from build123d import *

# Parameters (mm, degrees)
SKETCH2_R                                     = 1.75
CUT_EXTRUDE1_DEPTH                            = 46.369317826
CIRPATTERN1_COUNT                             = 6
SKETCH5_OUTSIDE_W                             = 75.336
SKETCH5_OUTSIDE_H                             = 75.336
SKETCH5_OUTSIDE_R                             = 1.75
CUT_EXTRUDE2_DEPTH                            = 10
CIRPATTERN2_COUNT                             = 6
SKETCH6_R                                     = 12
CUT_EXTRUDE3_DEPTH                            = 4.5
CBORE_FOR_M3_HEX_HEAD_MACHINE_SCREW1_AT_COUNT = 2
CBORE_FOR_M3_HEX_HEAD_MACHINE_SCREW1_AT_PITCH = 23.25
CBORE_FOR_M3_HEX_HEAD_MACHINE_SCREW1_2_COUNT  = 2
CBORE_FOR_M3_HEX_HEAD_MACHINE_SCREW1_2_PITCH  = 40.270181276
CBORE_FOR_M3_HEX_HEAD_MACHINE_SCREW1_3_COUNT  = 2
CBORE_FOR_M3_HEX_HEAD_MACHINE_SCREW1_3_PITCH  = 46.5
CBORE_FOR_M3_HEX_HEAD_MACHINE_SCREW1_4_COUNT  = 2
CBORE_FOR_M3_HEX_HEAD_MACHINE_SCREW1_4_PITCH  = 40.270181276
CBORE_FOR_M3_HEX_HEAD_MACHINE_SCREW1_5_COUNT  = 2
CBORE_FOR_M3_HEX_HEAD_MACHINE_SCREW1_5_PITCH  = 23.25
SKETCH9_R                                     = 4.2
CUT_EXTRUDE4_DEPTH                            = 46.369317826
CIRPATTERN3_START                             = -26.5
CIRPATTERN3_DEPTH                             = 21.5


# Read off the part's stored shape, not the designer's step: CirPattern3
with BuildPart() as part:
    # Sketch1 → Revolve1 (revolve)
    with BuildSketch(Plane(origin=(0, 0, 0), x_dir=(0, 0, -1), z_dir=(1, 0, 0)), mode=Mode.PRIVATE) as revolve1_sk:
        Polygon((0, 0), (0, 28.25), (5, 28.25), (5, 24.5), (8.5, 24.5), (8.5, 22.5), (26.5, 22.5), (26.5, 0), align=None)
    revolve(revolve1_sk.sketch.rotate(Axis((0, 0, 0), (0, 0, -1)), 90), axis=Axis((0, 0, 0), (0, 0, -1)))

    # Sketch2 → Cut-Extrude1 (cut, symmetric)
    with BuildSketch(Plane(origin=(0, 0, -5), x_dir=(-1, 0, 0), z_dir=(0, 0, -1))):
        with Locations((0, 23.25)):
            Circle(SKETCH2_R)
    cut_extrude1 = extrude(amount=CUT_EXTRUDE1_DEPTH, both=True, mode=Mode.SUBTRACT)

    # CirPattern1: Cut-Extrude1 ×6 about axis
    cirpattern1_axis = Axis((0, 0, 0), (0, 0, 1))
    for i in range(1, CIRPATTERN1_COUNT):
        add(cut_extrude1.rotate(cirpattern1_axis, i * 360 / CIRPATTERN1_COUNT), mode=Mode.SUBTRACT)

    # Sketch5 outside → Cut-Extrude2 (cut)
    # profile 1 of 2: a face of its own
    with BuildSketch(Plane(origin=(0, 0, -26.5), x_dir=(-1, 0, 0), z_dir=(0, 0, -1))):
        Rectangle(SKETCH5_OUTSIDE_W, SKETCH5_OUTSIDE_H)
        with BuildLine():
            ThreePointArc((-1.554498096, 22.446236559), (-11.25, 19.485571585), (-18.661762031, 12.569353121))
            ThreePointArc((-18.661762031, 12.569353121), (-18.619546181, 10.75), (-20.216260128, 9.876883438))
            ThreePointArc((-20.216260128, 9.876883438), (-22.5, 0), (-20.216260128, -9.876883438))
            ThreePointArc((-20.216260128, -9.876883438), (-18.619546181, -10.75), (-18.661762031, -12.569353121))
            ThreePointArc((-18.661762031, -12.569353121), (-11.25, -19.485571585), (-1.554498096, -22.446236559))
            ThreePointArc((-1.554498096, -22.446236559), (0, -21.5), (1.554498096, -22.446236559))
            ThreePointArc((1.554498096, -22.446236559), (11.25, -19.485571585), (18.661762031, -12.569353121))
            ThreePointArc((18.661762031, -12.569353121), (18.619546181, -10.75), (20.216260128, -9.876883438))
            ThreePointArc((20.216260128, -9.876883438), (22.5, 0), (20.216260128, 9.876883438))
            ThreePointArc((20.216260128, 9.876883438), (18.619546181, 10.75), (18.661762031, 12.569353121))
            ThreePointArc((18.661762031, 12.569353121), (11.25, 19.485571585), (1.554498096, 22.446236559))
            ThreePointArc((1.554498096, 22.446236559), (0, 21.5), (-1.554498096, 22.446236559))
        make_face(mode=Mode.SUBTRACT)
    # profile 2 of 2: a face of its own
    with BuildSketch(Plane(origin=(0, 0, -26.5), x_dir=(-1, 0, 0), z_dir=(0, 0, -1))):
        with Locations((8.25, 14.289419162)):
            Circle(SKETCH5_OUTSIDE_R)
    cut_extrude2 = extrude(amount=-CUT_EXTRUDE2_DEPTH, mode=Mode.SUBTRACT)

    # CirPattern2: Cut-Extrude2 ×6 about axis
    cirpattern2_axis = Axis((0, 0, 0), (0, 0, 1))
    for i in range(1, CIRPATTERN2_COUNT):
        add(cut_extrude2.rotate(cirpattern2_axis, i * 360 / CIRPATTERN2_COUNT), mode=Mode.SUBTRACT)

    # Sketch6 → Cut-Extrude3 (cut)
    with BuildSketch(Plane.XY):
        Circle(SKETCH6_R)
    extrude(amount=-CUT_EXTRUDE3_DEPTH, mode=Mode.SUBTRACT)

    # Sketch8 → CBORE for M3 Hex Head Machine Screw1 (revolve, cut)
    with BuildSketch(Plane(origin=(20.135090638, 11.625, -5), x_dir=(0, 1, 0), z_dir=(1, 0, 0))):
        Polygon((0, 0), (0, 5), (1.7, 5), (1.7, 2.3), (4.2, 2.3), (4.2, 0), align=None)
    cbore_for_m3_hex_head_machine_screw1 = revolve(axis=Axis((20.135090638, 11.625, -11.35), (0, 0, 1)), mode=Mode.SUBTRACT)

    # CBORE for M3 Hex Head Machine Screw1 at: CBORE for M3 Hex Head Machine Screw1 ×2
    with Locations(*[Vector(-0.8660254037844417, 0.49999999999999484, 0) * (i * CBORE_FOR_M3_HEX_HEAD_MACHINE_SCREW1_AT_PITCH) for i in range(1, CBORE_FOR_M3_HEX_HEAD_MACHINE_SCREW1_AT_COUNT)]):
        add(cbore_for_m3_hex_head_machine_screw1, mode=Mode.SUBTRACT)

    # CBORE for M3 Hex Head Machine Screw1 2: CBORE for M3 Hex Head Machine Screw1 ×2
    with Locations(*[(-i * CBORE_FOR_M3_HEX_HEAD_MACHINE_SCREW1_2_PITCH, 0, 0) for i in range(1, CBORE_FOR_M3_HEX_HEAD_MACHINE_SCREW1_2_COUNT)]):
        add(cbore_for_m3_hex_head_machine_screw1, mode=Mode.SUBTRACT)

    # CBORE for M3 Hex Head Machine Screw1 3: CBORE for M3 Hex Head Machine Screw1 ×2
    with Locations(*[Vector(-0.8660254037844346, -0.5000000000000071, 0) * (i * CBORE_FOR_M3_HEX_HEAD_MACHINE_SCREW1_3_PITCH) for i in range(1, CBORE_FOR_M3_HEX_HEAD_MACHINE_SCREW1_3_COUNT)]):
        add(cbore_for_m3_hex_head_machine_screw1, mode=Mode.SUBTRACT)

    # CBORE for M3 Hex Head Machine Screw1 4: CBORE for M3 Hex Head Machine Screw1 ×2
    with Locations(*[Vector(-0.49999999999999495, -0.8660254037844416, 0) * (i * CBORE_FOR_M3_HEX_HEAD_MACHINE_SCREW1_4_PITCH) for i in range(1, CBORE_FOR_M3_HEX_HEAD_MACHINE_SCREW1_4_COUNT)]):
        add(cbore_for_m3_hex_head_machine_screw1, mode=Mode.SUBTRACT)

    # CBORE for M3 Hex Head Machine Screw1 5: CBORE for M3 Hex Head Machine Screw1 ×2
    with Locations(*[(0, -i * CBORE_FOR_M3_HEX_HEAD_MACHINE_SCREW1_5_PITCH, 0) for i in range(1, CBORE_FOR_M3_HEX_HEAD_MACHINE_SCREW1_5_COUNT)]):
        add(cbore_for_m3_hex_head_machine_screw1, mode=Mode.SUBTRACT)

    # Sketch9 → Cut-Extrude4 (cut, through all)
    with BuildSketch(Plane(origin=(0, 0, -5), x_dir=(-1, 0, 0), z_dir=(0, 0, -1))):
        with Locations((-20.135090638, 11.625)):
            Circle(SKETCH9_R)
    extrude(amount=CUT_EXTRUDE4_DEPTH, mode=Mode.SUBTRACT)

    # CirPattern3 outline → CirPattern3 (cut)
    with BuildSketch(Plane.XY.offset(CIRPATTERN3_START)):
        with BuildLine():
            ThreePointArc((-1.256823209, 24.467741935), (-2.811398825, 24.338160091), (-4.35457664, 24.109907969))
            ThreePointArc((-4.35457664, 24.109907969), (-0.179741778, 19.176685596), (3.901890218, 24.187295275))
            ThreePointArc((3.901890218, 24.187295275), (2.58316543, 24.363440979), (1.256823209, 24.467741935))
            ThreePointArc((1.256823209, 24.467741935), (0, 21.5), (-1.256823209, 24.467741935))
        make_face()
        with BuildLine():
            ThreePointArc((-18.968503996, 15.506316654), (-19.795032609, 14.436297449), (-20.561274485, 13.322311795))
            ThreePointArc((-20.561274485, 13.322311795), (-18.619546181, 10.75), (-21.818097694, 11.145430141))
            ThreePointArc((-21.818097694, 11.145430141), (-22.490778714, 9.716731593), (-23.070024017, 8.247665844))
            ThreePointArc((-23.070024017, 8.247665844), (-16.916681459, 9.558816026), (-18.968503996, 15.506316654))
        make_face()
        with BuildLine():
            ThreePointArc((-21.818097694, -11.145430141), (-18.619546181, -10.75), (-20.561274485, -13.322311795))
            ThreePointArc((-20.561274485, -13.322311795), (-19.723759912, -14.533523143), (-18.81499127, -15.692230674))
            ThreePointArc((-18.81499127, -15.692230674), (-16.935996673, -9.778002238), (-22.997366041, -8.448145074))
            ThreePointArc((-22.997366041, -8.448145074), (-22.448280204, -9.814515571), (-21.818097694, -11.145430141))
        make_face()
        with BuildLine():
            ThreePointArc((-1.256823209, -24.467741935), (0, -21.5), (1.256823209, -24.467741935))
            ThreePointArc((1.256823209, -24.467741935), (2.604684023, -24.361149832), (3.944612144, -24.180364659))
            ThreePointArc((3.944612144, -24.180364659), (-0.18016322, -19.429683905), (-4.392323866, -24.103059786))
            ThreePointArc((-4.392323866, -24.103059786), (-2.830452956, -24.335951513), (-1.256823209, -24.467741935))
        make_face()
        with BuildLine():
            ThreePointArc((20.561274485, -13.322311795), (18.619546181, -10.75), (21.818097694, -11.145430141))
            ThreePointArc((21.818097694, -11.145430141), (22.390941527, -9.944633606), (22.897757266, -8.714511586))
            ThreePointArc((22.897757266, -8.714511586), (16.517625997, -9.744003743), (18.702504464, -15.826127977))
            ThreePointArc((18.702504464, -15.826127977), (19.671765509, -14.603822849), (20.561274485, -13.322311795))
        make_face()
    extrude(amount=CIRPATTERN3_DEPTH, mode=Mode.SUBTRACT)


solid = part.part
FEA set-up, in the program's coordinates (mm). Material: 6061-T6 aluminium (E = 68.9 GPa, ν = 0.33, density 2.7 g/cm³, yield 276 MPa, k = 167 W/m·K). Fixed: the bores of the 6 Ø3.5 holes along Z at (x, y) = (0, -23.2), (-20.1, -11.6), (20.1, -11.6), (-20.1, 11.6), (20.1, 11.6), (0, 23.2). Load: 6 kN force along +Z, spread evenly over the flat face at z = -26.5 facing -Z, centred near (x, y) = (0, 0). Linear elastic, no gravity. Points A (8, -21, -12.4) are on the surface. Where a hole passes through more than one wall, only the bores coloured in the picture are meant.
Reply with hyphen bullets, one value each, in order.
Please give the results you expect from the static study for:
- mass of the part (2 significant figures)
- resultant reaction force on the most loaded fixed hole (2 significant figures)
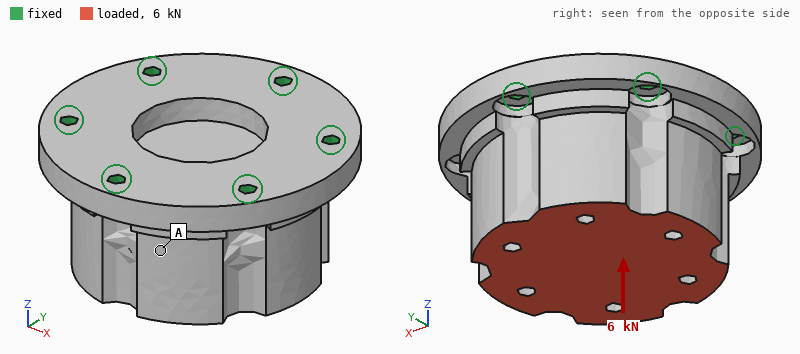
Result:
- 110 g
- 1.1 kN
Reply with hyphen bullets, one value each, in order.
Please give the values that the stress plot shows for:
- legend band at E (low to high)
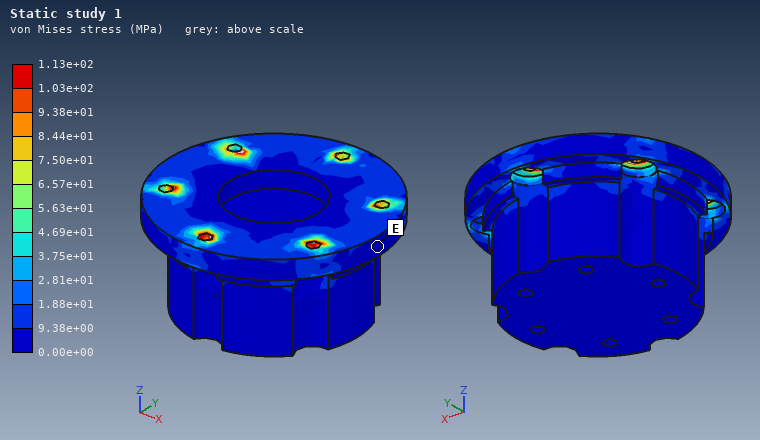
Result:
- 0.00e+00 to 9.38e+00 MPa
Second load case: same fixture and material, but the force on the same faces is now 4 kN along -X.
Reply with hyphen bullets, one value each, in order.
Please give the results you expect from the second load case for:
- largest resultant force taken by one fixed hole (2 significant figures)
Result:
- 1.5 kN
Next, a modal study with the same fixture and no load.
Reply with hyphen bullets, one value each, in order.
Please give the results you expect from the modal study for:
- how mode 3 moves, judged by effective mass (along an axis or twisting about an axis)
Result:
- along Z
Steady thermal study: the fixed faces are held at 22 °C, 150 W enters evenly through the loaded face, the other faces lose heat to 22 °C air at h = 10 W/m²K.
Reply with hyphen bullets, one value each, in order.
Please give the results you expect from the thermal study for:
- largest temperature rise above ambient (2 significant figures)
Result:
- 31 K
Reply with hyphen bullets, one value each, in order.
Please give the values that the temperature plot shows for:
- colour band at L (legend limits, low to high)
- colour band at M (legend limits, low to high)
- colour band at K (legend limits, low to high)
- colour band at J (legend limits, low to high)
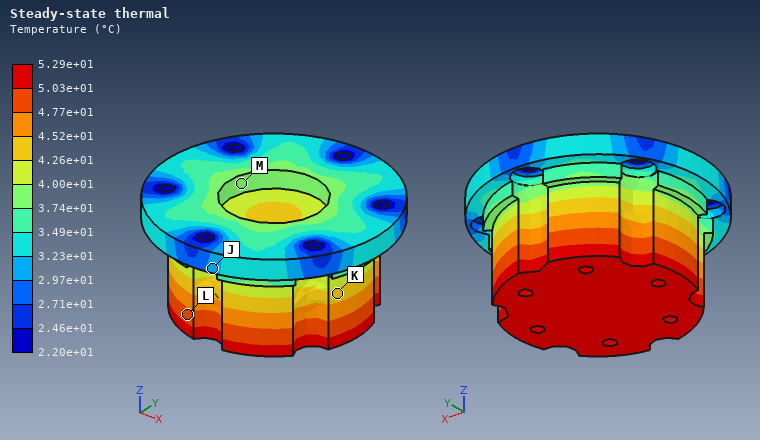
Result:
- 4.77e+01 to 5.03e+01 °C
- 3.74e+01 to 4.00e+01 °C
- 4.26e+01 to 4.52e+01 °C
- 2.97e+01 to 3.23e+01 °C
